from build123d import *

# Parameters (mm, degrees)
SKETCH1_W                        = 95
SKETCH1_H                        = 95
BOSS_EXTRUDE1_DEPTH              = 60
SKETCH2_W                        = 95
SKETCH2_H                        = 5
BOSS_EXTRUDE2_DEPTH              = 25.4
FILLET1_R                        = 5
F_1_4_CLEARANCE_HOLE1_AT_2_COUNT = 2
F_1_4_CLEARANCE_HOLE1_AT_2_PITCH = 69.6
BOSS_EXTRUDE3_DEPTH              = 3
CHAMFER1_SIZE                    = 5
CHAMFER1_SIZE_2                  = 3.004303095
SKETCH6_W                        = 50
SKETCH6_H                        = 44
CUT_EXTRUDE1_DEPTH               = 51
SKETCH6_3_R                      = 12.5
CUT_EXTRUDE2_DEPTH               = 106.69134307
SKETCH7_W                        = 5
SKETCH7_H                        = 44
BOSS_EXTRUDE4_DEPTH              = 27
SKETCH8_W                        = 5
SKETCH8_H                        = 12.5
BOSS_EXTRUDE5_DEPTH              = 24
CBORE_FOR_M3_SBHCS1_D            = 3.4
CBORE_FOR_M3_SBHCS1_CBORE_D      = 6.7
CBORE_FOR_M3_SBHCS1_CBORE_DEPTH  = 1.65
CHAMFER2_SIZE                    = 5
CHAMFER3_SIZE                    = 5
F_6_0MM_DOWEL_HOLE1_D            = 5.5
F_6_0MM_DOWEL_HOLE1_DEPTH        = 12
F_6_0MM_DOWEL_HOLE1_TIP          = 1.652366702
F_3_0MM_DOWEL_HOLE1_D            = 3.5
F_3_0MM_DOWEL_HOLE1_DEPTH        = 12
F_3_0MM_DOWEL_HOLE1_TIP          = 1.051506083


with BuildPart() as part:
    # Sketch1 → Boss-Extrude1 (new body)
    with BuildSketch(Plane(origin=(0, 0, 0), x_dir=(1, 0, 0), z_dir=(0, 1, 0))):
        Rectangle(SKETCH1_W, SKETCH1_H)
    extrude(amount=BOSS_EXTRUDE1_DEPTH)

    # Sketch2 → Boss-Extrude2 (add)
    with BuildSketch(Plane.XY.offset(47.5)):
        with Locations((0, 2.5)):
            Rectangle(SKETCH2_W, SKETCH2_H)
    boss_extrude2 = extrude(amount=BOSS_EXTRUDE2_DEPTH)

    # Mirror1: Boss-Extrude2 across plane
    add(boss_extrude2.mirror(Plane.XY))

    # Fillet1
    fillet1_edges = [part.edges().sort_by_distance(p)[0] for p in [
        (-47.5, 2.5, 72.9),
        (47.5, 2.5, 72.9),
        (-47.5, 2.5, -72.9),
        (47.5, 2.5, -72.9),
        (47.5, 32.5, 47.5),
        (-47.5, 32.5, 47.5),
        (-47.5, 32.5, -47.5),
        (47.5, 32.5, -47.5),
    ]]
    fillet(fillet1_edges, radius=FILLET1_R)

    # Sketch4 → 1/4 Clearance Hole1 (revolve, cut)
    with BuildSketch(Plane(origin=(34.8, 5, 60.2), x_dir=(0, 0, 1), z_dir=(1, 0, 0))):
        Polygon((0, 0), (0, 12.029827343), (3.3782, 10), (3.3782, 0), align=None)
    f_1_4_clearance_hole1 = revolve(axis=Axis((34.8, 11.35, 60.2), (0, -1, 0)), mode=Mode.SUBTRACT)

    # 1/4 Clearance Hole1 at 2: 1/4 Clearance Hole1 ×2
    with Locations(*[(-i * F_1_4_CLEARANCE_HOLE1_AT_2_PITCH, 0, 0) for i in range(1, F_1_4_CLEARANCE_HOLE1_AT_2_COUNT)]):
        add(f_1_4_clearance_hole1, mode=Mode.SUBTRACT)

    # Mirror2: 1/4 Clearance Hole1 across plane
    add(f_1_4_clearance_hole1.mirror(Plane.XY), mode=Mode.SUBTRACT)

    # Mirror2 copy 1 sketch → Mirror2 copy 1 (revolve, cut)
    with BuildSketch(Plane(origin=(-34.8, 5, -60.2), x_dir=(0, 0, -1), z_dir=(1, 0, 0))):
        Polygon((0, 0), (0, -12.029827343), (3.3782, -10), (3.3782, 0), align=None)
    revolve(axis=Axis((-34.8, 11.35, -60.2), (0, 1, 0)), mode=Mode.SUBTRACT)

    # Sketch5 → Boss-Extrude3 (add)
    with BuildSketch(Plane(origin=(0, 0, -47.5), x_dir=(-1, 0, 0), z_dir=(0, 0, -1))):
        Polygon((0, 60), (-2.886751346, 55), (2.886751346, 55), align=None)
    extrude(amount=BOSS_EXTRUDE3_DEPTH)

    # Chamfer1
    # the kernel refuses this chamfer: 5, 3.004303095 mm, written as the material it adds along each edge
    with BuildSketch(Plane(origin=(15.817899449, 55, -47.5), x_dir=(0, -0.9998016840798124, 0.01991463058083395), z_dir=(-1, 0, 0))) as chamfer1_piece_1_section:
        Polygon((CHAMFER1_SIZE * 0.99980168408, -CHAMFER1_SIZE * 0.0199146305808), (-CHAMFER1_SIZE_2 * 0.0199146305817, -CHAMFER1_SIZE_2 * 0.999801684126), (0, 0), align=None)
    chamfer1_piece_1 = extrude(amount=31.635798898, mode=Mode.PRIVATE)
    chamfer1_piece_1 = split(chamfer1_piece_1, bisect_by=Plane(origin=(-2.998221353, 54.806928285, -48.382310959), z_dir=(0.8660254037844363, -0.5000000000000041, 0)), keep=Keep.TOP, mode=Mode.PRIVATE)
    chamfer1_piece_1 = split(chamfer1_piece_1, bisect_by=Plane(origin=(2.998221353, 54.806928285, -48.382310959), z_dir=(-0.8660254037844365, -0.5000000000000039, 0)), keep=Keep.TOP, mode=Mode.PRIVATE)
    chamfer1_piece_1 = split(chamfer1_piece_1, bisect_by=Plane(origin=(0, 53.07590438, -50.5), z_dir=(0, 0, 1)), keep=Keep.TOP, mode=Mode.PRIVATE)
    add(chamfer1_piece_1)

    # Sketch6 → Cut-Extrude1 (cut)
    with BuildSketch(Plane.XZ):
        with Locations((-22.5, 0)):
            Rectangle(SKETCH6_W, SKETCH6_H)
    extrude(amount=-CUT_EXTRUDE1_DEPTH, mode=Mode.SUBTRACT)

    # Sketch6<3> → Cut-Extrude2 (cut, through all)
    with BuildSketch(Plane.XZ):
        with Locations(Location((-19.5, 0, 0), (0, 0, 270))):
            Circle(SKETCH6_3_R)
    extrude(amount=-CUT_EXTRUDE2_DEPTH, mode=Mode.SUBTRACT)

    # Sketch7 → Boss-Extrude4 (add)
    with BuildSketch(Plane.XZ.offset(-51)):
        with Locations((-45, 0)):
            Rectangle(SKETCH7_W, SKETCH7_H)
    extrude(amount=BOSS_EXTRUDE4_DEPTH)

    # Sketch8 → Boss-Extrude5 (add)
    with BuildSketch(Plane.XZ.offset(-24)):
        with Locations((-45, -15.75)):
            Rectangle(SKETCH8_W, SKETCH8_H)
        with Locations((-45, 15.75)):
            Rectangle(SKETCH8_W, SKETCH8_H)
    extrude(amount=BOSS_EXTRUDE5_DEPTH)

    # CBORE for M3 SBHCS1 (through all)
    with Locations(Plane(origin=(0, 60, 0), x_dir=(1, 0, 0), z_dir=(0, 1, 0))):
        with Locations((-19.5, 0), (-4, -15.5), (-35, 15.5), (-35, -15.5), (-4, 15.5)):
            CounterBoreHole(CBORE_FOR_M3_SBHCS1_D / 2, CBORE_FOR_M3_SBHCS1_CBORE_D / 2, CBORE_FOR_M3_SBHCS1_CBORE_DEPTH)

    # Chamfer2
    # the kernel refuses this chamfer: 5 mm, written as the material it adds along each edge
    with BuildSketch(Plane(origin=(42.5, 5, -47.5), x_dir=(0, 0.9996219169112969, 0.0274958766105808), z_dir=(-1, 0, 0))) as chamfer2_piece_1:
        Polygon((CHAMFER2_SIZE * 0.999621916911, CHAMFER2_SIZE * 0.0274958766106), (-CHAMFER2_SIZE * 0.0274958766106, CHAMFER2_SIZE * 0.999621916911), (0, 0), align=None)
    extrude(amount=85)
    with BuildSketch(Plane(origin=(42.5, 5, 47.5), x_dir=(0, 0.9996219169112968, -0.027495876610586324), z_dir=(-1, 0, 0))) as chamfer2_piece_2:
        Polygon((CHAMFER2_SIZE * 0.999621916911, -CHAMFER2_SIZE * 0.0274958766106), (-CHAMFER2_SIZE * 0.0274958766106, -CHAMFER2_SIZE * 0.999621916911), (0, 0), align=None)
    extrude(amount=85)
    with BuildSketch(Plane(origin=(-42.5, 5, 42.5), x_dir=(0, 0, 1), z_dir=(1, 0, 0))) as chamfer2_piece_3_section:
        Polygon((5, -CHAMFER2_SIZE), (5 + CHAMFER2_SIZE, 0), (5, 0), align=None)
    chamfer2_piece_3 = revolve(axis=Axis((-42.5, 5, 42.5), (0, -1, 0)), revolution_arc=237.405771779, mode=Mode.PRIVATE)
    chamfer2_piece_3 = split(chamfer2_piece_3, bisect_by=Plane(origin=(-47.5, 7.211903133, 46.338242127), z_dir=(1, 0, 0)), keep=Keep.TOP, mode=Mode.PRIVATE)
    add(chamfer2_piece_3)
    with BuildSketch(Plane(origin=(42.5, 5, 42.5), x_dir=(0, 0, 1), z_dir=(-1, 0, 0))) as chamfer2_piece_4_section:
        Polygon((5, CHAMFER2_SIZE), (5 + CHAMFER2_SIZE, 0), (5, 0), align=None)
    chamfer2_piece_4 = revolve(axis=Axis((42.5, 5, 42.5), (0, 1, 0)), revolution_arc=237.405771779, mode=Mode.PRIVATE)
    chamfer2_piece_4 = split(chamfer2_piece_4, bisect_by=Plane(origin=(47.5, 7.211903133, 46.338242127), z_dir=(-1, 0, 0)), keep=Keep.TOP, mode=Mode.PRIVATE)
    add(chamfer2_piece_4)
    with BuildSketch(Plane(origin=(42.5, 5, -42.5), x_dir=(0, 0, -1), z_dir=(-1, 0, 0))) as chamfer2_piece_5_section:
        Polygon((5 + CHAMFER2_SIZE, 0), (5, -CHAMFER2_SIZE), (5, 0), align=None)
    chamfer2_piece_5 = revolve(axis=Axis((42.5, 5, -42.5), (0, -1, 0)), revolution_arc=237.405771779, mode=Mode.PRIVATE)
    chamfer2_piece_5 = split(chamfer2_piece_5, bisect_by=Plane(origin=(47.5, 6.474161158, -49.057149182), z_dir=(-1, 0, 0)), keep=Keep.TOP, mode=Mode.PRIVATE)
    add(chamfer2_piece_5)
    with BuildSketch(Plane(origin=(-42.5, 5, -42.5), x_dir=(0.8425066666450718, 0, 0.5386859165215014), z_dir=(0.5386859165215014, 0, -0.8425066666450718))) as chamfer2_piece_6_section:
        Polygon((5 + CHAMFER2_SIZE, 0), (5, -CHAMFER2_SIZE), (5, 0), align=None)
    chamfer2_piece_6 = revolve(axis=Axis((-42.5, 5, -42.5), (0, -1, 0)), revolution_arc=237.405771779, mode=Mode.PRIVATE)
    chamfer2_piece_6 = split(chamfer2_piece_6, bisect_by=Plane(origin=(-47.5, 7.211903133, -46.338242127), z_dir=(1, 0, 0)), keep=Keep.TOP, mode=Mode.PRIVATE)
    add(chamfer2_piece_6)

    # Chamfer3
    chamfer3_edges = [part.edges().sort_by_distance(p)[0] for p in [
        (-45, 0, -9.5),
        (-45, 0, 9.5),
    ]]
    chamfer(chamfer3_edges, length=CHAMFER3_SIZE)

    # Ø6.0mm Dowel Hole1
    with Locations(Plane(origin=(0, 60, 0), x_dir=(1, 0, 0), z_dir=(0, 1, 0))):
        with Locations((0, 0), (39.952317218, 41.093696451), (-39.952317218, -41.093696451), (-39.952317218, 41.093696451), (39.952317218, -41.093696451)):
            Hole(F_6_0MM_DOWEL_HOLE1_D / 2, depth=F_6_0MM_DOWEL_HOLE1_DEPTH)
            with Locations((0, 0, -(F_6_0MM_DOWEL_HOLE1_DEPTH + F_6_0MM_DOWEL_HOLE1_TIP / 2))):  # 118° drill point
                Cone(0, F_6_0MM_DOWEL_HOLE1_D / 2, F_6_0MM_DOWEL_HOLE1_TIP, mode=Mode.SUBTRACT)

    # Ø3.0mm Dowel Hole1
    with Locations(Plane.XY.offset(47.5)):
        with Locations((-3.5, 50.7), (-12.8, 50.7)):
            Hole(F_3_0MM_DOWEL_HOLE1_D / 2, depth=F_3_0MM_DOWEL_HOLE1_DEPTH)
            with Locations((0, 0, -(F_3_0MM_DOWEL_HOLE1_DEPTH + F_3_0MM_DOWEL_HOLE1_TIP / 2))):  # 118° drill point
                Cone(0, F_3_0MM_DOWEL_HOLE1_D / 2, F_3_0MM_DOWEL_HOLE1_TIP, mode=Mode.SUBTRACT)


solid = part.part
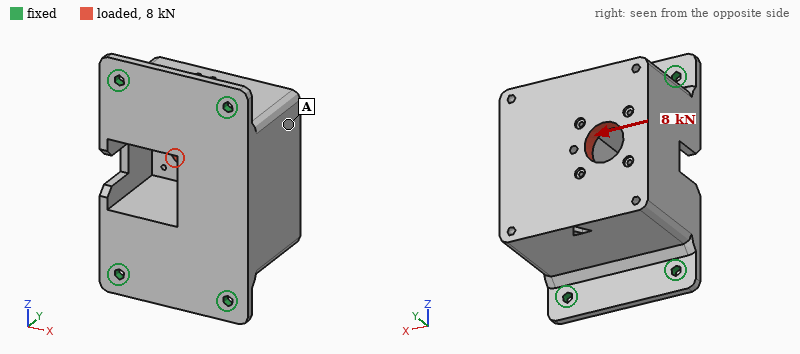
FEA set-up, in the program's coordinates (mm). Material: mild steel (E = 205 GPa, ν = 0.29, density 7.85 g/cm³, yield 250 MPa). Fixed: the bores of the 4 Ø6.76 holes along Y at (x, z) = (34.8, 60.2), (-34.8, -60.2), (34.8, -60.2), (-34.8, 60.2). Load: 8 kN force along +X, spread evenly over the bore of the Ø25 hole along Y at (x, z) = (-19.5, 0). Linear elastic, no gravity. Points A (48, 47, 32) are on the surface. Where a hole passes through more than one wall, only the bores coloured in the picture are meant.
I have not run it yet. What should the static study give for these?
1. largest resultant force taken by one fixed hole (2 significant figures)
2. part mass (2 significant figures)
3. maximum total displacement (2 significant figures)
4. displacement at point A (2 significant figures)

4.4 kN
3.6 kg
29 µm
23 µm
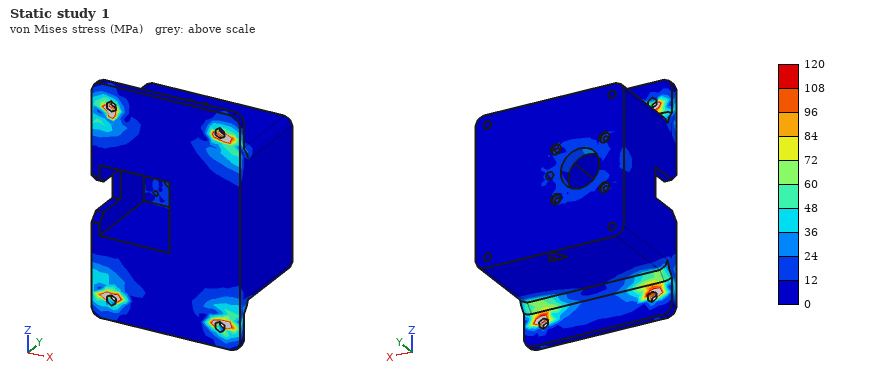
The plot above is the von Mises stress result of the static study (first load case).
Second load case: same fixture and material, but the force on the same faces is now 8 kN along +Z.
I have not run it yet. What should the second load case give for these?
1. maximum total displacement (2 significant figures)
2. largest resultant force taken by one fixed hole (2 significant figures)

13 µm
2.9 kN
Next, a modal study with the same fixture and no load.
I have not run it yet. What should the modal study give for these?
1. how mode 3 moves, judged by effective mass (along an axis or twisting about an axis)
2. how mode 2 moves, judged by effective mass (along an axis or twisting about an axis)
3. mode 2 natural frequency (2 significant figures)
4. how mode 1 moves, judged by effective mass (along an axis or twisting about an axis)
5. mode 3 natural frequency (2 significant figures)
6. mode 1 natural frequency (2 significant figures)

along Z
along Y
2800 Hz
along X
3400 Hz
2200 Hz
